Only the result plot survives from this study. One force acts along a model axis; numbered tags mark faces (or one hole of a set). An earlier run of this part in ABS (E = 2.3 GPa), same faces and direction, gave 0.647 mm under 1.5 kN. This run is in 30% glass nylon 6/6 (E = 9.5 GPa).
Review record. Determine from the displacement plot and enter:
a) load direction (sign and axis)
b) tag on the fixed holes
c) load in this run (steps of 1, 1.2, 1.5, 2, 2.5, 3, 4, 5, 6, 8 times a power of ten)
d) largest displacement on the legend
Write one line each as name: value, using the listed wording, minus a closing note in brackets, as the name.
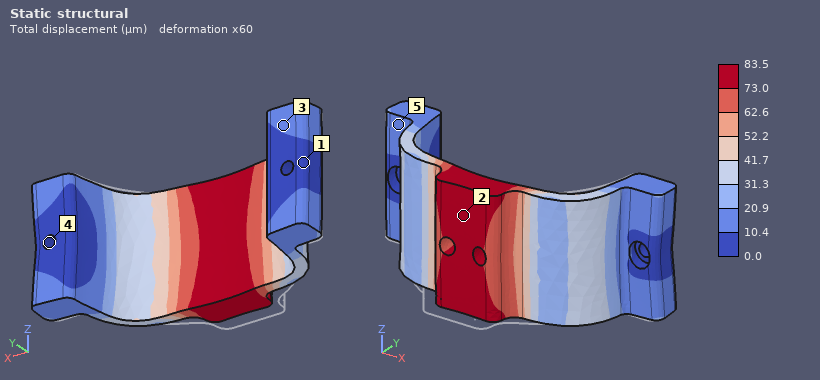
load direction: +Y
tag on the fixed holes: 4
load in this run: 800 N
largest displacement on the legend: 83.5 µm
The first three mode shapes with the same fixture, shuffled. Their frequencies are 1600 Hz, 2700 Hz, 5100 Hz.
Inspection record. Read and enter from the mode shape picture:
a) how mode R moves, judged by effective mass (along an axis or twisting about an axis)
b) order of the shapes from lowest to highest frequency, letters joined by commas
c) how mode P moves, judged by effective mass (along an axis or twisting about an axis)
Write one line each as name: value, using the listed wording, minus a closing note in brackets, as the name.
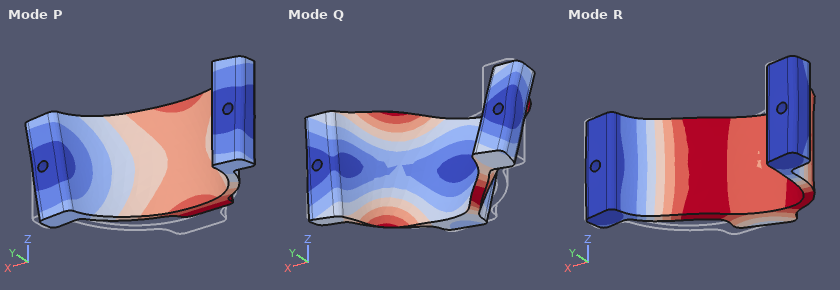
how mode R moves, judged by effective mass: along X
order of the shapes from lowest to highest frequency, letters joined by commas: P, R, Q
how mode P moves, judged by effective mass: along Z
